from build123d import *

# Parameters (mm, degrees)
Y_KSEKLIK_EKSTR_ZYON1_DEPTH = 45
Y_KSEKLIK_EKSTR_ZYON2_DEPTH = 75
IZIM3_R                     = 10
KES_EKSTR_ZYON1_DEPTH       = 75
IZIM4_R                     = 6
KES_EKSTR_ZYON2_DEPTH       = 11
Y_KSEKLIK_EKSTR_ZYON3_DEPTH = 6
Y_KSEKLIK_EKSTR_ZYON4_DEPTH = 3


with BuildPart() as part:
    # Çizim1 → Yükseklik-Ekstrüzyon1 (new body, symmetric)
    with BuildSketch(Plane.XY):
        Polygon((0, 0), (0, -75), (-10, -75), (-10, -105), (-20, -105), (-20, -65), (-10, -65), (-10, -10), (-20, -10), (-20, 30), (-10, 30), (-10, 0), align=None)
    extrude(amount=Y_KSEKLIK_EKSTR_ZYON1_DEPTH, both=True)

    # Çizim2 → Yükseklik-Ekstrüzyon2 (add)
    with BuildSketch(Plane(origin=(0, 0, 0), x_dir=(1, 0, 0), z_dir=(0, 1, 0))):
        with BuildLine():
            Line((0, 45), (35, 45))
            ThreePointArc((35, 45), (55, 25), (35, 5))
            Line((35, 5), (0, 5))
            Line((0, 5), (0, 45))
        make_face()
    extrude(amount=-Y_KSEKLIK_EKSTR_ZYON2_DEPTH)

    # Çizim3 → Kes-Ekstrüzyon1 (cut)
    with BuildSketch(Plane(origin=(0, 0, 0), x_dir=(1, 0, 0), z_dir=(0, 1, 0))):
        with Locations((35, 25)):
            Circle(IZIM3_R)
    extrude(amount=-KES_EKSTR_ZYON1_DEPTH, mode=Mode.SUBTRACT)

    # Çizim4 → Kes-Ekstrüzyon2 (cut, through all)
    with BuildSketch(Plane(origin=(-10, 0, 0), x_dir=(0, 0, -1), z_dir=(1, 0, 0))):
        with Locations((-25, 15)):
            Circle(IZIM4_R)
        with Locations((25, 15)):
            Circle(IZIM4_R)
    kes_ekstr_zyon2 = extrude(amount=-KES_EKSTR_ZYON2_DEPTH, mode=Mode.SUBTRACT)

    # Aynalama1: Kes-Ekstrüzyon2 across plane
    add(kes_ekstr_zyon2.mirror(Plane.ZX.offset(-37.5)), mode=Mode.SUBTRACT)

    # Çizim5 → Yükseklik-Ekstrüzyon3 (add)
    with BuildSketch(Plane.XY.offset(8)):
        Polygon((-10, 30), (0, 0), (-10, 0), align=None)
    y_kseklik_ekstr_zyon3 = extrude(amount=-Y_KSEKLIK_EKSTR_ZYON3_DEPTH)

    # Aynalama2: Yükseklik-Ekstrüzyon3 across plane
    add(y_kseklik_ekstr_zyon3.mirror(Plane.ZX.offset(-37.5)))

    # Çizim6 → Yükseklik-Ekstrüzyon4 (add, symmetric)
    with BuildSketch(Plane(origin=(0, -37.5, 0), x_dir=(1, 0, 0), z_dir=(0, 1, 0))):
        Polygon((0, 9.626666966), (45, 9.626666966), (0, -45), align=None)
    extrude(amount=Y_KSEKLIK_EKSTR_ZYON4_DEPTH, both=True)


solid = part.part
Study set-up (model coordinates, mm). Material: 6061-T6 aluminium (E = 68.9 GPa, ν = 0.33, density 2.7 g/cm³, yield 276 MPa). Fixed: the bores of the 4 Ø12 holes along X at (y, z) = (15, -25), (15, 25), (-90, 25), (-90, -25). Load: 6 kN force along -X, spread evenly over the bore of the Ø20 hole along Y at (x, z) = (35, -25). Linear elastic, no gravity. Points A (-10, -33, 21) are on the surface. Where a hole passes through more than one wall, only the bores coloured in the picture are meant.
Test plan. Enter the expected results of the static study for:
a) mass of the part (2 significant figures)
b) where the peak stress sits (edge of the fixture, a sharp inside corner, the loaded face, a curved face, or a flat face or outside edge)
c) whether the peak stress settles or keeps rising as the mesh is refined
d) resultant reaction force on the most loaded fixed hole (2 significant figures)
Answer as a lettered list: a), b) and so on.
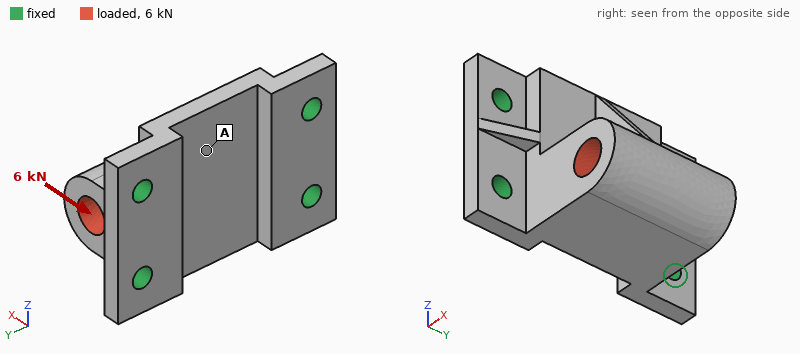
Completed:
a) 730 g
b) edge of the fixture
c) keeps rising
d) 3.5 kN
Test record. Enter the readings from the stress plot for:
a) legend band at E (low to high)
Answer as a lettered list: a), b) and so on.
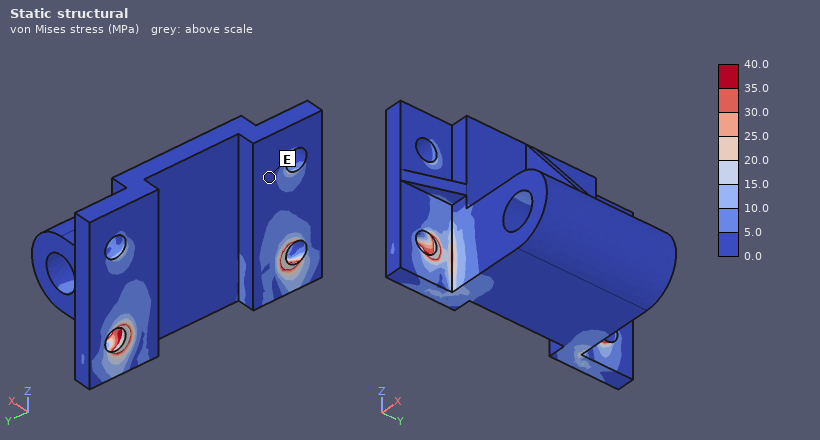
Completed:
a) 0.0 to 5.0 MPa
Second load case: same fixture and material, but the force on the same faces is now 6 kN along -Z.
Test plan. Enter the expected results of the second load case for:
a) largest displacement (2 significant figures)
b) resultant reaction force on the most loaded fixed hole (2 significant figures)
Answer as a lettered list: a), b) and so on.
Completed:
a) 83 µm
b) 4.9 kN
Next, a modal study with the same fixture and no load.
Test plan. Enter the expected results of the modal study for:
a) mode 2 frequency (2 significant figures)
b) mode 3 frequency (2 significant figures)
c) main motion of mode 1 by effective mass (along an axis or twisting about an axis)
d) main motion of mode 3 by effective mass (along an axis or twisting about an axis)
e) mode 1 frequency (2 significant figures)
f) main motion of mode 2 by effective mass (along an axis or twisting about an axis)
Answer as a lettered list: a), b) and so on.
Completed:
a) 5000 Hz
b) 5200 Hz
c) along Z
d) along X
e) 2900 Hz
f) along Y
